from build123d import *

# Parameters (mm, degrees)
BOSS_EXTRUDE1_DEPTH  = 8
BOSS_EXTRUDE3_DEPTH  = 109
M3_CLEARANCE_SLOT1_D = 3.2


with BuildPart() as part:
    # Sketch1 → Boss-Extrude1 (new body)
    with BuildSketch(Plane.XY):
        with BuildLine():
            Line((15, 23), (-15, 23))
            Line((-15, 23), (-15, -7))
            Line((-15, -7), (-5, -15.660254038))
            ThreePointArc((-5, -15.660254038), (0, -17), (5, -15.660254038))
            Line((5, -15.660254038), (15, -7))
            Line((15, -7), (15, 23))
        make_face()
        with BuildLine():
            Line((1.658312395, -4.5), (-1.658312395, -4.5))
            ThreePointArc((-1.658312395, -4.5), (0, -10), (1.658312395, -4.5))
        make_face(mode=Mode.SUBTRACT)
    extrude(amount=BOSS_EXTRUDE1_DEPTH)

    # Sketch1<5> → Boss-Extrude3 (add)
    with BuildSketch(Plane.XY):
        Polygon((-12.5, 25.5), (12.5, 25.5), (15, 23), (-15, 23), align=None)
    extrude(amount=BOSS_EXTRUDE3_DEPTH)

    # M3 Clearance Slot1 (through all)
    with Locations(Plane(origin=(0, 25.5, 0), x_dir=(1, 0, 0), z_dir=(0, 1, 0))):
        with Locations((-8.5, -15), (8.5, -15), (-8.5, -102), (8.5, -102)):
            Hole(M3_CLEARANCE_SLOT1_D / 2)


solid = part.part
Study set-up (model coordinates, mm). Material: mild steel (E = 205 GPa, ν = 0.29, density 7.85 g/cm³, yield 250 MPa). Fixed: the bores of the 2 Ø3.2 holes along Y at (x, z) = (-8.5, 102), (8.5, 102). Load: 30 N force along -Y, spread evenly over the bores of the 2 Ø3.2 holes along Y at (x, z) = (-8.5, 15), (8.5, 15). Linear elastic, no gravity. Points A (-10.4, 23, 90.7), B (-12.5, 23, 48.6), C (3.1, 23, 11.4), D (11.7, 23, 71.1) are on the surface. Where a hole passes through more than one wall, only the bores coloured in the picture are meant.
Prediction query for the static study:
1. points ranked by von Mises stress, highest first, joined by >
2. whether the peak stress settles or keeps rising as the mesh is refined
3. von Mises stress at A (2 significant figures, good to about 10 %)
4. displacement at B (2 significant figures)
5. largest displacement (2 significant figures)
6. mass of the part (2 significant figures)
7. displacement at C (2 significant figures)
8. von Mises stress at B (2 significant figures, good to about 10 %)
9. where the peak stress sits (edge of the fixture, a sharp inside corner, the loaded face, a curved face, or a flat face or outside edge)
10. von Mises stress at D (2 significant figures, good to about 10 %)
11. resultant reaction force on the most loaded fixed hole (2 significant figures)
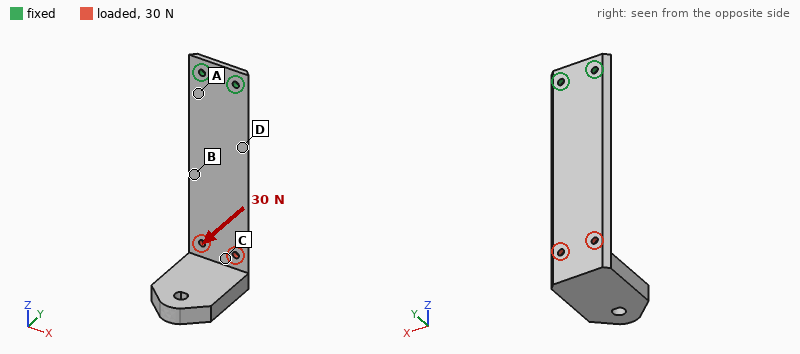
A > D > B > C
keeps rising
76 MPa
0.39 mm
1.3 mm
120 g
0.94 mm
34 MPa
edge of the fixture
57 MPa
21 N
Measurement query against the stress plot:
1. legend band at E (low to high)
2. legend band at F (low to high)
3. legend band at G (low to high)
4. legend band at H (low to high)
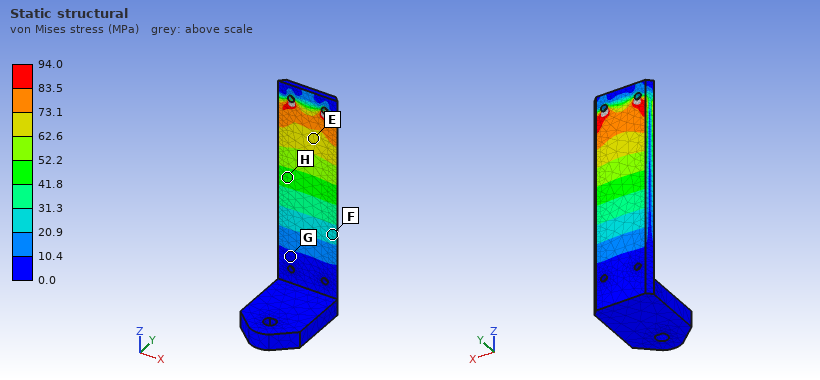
62.6 to 73.1 MPa
20.9 to 31.3 MPa
0.0 to 10.4 MPa
41.8 to 52.2 MPa
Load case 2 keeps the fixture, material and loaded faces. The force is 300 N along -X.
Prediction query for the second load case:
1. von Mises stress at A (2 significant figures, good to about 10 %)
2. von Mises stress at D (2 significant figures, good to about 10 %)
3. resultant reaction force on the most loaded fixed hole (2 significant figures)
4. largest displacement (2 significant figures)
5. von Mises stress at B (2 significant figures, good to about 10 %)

53 MPa
45 MPa
1.4 kN
0.11 mm
29 MPa
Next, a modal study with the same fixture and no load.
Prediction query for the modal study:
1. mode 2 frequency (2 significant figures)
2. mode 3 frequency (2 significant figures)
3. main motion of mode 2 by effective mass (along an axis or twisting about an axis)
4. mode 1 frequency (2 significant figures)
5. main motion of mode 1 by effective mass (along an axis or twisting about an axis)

280 Hz
470 Hz
along X
82 Hz
along Y
